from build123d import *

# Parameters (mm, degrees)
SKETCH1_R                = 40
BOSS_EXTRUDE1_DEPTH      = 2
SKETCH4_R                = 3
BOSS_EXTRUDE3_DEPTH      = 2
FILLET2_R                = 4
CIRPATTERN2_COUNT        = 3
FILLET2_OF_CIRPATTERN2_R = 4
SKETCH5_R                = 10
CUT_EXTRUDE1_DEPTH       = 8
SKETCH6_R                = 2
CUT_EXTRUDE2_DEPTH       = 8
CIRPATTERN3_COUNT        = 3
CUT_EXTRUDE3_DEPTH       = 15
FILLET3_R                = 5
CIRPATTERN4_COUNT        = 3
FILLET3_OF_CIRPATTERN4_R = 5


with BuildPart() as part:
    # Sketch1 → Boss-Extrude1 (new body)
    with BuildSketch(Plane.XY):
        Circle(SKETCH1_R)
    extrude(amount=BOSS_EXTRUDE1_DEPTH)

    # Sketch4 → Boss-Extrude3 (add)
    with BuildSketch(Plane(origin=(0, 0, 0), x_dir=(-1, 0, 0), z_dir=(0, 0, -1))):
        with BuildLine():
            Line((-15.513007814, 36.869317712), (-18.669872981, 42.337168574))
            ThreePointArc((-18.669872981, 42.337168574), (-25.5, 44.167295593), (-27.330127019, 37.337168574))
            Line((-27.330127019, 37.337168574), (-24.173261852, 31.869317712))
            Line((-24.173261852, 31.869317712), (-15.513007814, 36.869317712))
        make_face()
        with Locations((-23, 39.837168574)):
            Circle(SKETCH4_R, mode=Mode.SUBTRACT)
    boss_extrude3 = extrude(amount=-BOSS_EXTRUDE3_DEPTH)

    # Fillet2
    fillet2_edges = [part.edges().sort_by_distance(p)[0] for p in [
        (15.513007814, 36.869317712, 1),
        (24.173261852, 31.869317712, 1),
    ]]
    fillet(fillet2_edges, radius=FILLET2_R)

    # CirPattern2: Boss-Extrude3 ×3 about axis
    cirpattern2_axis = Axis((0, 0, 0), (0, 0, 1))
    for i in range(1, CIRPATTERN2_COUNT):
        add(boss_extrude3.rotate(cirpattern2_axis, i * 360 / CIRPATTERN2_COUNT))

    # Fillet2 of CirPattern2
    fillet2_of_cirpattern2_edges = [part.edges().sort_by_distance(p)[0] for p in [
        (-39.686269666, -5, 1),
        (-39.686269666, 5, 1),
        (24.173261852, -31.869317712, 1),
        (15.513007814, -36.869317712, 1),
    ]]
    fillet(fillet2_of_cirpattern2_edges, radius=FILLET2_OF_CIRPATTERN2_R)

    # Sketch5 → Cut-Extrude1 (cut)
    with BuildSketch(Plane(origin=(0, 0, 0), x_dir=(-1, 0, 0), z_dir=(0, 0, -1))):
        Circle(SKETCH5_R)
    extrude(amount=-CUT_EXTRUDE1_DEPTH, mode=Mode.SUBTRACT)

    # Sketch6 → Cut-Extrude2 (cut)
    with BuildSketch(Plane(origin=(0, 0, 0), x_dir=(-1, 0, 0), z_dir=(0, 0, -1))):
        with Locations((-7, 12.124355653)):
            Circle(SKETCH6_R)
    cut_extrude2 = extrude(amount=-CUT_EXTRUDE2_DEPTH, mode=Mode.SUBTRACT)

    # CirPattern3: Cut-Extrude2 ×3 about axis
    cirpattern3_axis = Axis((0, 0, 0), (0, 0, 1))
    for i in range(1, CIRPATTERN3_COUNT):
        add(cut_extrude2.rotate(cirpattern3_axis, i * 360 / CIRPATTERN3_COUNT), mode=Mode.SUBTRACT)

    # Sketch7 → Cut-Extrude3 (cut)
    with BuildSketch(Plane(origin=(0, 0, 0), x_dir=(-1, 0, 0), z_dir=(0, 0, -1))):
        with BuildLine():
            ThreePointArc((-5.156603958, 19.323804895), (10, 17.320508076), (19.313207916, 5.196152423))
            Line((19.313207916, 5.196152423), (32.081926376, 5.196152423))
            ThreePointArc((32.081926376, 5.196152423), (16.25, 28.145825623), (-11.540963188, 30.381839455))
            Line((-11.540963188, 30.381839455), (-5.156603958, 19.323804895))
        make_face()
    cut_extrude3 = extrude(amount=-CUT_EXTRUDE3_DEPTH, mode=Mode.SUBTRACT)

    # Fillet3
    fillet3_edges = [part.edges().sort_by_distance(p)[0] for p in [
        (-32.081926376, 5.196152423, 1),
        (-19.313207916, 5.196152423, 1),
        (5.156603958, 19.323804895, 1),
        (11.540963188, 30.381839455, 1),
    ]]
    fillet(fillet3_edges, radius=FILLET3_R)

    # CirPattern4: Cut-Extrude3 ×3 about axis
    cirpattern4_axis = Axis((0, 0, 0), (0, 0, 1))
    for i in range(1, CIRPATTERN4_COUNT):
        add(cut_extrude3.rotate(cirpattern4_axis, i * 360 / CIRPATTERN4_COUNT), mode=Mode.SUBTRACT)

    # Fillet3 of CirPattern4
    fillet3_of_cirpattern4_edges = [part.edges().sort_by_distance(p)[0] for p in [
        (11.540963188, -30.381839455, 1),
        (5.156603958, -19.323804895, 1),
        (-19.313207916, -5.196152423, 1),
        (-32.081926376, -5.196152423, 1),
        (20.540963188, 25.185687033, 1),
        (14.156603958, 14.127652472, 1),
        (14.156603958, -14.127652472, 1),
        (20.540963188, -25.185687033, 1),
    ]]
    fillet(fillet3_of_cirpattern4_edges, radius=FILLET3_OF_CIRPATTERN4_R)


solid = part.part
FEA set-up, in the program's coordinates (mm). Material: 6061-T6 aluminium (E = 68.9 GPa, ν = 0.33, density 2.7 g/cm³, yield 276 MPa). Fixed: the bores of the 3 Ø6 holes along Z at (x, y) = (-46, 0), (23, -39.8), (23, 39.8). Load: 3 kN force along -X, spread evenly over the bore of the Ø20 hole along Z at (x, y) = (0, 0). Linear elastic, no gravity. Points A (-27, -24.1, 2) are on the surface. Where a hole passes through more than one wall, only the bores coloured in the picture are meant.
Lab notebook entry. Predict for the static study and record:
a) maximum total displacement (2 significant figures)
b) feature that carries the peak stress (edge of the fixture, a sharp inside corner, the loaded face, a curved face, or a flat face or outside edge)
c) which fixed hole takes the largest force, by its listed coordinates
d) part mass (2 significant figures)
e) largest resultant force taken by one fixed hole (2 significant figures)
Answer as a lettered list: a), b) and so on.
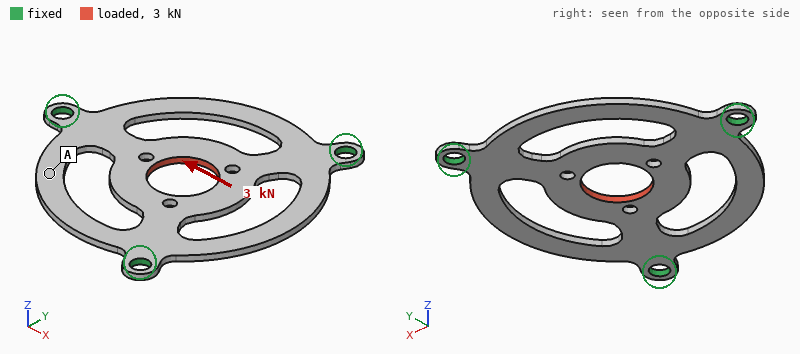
a) 91 µm
b) a curved face
c) (-46, 0)
d) 18 g
e) 1.6 kN
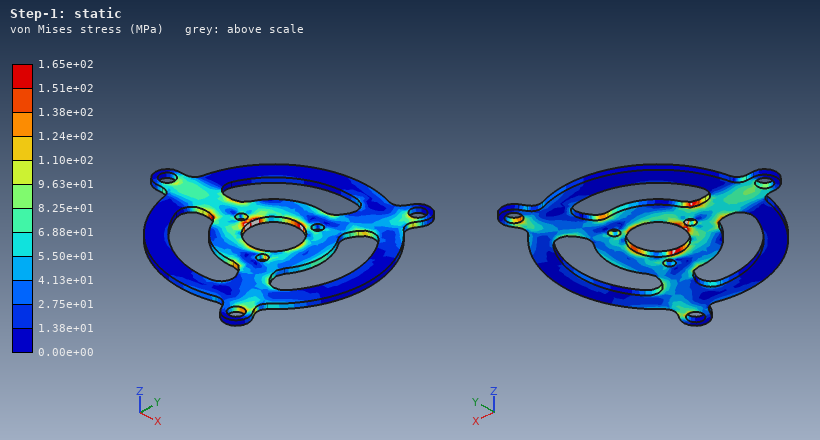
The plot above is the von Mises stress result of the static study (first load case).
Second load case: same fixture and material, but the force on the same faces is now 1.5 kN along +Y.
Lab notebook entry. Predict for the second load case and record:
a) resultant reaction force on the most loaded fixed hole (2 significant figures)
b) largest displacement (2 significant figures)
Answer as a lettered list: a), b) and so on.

a) 690 N
b) 44 µm
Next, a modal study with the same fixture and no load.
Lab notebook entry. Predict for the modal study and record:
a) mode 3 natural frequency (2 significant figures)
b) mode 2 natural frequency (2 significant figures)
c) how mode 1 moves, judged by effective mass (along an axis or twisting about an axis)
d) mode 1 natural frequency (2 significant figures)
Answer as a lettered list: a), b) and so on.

a) 1600 Hz
b) 1600 Hz
c) along Z
d) 1500 Hz
